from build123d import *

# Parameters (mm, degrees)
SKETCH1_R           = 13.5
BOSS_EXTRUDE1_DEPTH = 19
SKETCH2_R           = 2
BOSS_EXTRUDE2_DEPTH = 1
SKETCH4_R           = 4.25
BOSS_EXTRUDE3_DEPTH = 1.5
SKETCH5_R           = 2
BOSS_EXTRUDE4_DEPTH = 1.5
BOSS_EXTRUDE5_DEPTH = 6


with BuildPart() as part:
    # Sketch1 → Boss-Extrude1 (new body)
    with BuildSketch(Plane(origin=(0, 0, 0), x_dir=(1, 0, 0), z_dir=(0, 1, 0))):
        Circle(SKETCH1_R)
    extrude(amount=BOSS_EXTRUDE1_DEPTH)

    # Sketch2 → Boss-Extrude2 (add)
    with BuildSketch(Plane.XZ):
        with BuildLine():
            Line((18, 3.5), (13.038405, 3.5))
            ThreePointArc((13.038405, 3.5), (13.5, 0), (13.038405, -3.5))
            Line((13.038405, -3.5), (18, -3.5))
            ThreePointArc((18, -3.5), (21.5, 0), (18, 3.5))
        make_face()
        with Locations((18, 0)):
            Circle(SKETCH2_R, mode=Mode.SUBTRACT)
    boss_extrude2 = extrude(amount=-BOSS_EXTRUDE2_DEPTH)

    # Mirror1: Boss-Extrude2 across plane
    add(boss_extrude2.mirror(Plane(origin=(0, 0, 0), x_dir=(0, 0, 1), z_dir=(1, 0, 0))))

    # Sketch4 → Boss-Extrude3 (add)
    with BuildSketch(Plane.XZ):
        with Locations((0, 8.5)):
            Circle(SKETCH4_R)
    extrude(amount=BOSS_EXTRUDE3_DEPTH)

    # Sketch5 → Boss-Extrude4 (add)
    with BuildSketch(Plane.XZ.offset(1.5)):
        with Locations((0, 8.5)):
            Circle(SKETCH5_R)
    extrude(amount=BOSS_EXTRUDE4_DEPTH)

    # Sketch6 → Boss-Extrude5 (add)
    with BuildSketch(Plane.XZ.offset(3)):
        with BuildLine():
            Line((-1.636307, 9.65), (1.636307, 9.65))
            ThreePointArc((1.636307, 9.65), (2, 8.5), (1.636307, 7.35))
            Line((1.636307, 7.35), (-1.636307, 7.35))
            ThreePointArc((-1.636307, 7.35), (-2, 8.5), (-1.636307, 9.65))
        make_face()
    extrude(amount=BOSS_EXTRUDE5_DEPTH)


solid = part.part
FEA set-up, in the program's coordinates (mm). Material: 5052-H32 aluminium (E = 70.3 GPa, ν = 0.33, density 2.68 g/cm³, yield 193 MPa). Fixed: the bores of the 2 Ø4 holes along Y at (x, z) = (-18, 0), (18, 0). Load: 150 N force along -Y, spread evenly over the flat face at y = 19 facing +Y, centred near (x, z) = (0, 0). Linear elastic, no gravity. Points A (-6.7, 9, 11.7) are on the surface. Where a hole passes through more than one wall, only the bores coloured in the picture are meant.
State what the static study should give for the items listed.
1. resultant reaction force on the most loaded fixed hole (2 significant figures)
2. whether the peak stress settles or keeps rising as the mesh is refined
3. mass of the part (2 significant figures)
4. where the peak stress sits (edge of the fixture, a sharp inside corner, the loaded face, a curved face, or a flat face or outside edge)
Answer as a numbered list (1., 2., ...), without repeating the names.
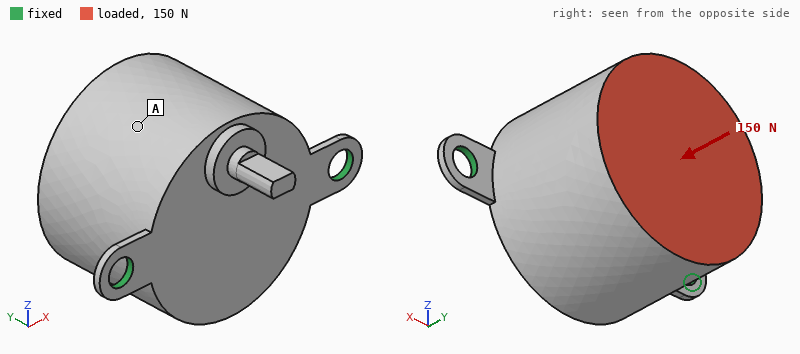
1. 87 N
2. keeps rising
3. 30 g
4. edge of the fixture
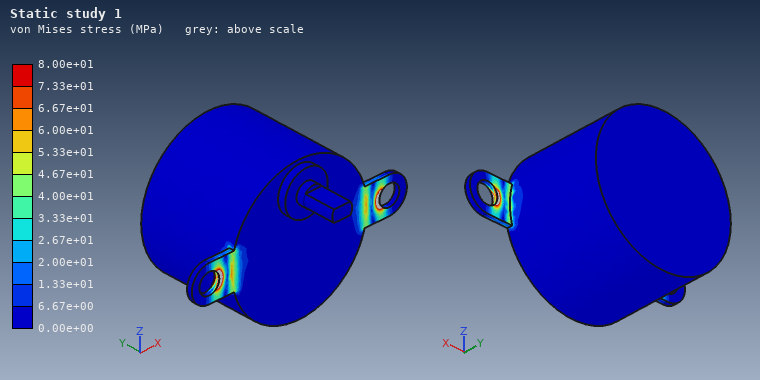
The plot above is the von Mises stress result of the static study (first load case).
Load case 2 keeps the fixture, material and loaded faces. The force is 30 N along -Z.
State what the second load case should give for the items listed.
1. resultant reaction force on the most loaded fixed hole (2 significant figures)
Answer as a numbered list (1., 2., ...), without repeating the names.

1. 15 N
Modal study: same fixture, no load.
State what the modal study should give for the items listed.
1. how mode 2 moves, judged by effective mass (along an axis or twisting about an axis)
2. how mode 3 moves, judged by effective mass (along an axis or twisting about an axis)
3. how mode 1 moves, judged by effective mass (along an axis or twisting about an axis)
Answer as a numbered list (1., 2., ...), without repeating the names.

1. along Y
2. along X
3. along Z
